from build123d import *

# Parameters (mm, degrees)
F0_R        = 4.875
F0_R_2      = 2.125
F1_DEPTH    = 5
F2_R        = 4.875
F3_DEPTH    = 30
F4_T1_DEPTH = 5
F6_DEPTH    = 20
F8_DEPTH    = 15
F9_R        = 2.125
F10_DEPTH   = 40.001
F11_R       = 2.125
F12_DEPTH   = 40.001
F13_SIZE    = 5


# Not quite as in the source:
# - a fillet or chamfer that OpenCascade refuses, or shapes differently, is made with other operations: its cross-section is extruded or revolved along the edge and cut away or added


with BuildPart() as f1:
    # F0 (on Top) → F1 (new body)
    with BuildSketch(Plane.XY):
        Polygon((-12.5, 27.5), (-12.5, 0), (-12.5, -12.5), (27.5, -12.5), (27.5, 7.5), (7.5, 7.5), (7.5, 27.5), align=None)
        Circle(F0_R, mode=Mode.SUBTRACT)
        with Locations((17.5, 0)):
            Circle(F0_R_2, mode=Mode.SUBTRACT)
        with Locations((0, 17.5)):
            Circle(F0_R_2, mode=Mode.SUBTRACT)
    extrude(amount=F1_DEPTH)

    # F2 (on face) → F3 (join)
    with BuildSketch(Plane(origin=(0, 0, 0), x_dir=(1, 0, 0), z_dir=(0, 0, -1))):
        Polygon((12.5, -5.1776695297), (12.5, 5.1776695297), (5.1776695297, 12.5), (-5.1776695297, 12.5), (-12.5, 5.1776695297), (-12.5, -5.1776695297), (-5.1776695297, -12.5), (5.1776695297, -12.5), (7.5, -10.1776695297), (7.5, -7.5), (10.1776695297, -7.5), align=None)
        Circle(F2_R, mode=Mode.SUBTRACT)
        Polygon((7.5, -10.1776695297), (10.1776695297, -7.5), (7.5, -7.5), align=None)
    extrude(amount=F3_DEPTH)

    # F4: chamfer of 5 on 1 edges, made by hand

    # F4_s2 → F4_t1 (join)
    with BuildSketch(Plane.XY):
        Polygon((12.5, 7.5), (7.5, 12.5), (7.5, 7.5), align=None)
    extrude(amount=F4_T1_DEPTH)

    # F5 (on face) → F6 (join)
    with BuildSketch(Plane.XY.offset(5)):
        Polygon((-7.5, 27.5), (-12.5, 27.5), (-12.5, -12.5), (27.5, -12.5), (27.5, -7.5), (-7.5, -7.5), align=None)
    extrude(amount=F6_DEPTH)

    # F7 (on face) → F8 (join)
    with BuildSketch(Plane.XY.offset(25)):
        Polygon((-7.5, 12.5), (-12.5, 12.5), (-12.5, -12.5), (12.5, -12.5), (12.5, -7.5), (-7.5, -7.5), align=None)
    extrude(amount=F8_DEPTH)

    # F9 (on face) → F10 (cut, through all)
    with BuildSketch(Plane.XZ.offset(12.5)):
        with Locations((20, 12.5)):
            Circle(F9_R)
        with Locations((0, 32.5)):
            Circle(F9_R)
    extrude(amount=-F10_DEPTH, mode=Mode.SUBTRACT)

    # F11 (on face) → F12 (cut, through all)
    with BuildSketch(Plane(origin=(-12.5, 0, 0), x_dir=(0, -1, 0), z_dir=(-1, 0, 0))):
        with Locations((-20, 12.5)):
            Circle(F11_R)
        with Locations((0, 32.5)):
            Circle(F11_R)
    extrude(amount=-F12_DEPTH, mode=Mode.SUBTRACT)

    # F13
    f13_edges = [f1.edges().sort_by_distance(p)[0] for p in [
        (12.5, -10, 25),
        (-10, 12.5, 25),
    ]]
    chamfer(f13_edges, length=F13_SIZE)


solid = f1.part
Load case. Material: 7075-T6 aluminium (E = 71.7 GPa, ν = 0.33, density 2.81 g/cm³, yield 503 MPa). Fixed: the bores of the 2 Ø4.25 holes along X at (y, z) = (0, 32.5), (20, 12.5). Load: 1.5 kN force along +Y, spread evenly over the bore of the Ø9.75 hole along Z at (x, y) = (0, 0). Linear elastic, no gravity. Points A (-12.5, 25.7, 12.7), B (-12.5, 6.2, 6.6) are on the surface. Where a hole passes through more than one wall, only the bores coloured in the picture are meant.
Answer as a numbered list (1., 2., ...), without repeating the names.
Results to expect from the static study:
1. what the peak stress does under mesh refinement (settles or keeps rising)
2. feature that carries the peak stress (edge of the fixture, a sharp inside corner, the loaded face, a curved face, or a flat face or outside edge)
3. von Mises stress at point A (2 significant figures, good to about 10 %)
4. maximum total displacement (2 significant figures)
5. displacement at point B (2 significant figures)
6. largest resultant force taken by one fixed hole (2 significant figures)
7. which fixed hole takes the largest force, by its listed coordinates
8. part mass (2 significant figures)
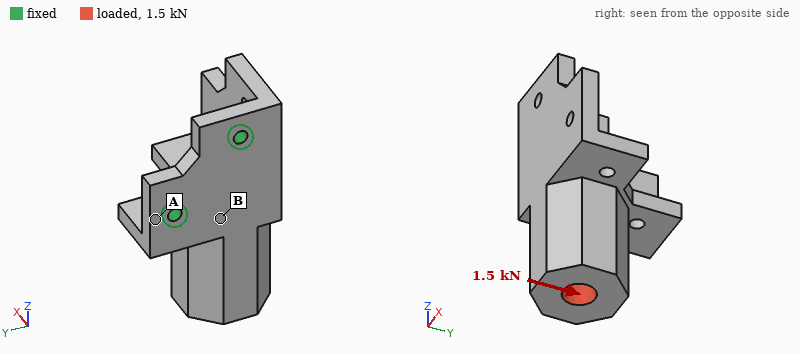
1. keeps rising
2. edge of the fixture
3. 35 MPa
4. 0.16 mm
5. 0.026 mm
6. 2.3 kN
7. (20, 12.5)
8. 83 g
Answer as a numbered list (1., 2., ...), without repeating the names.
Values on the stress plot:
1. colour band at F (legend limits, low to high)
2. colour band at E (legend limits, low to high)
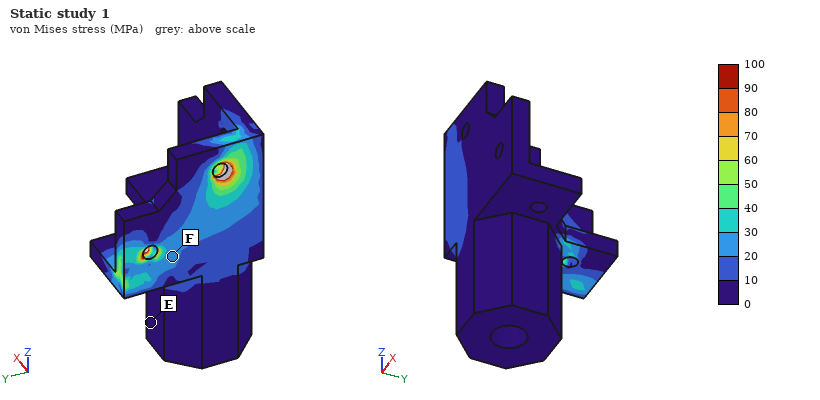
1. 20 to 30 MPa
2. 0 to 10 MPa
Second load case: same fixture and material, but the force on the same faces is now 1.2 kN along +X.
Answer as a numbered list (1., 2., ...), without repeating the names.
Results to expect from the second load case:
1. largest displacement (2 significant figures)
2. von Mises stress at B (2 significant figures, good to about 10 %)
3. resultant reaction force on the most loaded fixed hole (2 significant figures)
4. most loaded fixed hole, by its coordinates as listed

1. 0.53 mm
2. 48 MPa
3. 1.1 kN
4. (20, 12.5)
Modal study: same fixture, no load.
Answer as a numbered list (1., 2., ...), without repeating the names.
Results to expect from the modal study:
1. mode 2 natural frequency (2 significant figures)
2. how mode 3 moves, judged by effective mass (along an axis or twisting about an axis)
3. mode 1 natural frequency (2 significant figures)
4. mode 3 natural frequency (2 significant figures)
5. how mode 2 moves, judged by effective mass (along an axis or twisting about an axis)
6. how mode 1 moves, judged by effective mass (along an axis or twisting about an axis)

1. 4200 Hz
2. along Y
3. 1200 Hz
4. 5400 Hz
5. along Y
6. along X
